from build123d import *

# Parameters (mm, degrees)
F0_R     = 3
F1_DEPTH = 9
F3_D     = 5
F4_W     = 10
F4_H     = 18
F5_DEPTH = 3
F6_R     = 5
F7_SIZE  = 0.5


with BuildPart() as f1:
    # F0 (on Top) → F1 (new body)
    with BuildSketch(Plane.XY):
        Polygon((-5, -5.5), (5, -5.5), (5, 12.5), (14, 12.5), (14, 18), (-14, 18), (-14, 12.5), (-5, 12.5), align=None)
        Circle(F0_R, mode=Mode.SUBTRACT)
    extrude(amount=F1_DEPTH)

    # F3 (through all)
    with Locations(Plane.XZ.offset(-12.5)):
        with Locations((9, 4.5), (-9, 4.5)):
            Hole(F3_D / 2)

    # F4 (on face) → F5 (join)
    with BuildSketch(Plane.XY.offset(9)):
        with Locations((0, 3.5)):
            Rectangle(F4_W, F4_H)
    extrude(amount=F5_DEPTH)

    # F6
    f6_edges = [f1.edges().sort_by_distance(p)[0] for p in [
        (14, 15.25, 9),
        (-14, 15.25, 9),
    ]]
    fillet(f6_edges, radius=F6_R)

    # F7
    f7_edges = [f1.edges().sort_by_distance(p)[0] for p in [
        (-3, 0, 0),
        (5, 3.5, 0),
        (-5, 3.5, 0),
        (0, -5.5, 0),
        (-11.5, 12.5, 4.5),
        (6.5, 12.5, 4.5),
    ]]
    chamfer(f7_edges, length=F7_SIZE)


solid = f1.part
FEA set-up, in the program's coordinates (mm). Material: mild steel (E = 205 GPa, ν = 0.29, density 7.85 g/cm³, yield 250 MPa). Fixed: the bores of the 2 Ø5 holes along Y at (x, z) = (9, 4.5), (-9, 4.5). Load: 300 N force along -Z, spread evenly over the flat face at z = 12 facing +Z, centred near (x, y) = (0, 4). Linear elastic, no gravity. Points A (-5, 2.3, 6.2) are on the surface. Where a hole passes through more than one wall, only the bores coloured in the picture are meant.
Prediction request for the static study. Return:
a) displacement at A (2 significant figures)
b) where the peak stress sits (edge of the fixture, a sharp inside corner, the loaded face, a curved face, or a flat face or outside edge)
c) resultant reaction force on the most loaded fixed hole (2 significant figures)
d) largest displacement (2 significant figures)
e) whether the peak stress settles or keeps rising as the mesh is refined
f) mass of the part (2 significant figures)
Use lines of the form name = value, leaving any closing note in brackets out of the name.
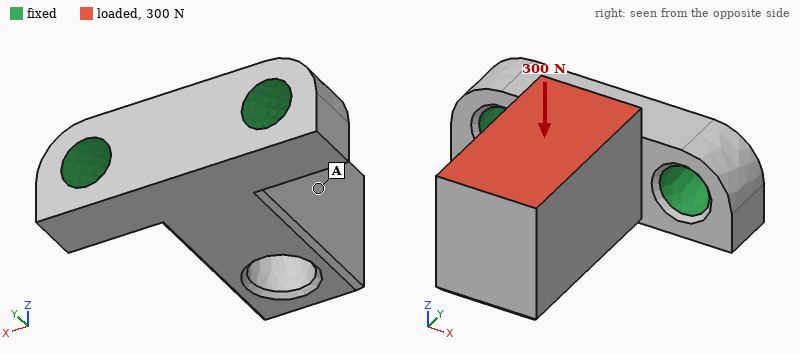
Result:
displacement at A = 4.7 µm
where the peak stress sits = edge of the fixture
resultant reaction force on the most loaded fixed hole = 150 N
largest displacement = 8.2 µm
whether the peak stress settles or keeps rising as the mesh is refined = keeps rising
mass of the part = 24 g
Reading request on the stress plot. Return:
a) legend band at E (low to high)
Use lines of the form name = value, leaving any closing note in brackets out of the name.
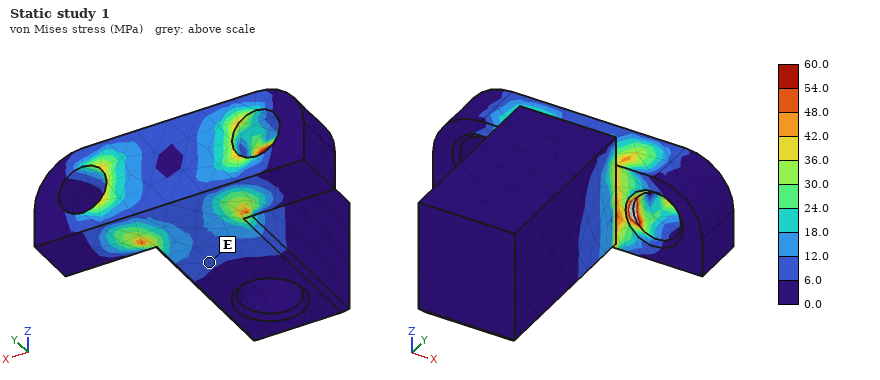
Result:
legend band at E = 6.0 to 12.0 MPa
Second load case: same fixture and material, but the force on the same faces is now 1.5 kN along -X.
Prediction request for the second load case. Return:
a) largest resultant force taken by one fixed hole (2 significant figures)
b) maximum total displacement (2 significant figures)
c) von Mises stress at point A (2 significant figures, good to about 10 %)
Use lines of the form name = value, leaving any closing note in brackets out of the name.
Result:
largest resultant force taken by one fixed hole = 1.7 kN
maximum total displacement = 21 µm
von Mises stress at point A = 32 MPa
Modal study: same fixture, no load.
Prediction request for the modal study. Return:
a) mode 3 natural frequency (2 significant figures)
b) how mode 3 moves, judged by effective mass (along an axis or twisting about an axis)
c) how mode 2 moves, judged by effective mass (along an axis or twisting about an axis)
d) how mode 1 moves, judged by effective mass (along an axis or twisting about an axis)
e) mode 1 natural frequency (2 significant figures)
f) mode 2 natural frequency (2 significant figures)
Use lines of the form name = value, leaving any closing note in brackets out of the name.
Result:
mode 3 natural frequency = 33 kHz
how mode 3 moves, judged by effective mass = twisting about Y
how mode 2 moves, judged by effective mass = along X
how mode 1 moves, judged by effective mass = along Z
mode 1 natural frequency = 9800 Hz
mode 2 natural frequency = 15 kHz
